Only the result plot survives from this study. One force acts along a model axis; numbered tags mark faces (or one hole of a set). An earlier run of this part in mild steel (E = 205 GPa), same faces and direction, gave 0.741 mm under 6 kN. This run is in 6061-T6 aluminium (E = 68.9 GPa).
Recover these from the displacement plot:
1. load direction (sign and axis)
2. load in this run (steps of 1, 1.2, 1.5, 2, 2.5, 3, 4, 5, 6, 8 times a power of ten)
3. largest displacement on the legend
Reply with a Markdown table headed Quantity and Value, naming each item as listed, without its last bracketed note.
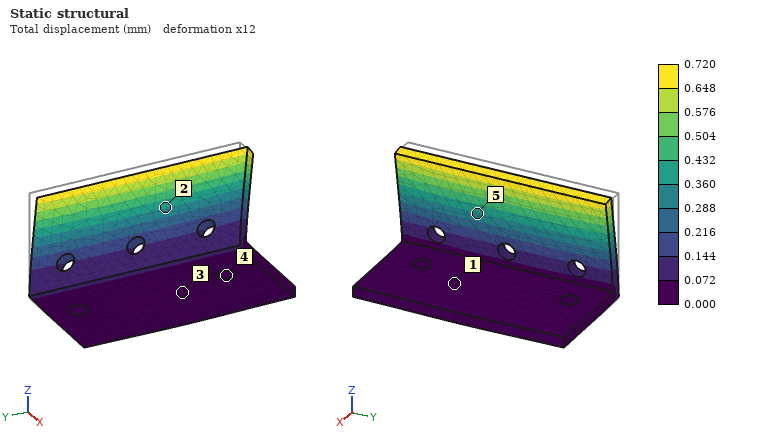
| Quantity | Value |
|---|---|
| load direction | +X |
| load in this run | 2 kN |
| largest displacement on the legend | 0.720 mm |
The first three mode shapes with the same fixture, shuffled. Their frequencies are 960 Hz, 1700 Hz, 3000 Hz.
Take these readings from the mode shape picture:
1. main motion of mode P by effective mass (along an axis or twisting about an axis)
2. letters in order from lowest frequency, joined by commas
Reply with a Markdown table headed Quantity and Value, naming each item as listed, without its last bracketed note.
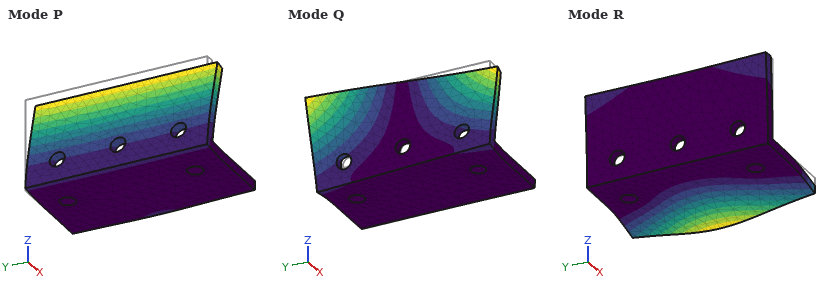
| Quantity | Value |
|---|---|
| main motion of mode P by effective mass | along X |
| letters in order from lowest frequency, joined by commas | P, Q, R |
